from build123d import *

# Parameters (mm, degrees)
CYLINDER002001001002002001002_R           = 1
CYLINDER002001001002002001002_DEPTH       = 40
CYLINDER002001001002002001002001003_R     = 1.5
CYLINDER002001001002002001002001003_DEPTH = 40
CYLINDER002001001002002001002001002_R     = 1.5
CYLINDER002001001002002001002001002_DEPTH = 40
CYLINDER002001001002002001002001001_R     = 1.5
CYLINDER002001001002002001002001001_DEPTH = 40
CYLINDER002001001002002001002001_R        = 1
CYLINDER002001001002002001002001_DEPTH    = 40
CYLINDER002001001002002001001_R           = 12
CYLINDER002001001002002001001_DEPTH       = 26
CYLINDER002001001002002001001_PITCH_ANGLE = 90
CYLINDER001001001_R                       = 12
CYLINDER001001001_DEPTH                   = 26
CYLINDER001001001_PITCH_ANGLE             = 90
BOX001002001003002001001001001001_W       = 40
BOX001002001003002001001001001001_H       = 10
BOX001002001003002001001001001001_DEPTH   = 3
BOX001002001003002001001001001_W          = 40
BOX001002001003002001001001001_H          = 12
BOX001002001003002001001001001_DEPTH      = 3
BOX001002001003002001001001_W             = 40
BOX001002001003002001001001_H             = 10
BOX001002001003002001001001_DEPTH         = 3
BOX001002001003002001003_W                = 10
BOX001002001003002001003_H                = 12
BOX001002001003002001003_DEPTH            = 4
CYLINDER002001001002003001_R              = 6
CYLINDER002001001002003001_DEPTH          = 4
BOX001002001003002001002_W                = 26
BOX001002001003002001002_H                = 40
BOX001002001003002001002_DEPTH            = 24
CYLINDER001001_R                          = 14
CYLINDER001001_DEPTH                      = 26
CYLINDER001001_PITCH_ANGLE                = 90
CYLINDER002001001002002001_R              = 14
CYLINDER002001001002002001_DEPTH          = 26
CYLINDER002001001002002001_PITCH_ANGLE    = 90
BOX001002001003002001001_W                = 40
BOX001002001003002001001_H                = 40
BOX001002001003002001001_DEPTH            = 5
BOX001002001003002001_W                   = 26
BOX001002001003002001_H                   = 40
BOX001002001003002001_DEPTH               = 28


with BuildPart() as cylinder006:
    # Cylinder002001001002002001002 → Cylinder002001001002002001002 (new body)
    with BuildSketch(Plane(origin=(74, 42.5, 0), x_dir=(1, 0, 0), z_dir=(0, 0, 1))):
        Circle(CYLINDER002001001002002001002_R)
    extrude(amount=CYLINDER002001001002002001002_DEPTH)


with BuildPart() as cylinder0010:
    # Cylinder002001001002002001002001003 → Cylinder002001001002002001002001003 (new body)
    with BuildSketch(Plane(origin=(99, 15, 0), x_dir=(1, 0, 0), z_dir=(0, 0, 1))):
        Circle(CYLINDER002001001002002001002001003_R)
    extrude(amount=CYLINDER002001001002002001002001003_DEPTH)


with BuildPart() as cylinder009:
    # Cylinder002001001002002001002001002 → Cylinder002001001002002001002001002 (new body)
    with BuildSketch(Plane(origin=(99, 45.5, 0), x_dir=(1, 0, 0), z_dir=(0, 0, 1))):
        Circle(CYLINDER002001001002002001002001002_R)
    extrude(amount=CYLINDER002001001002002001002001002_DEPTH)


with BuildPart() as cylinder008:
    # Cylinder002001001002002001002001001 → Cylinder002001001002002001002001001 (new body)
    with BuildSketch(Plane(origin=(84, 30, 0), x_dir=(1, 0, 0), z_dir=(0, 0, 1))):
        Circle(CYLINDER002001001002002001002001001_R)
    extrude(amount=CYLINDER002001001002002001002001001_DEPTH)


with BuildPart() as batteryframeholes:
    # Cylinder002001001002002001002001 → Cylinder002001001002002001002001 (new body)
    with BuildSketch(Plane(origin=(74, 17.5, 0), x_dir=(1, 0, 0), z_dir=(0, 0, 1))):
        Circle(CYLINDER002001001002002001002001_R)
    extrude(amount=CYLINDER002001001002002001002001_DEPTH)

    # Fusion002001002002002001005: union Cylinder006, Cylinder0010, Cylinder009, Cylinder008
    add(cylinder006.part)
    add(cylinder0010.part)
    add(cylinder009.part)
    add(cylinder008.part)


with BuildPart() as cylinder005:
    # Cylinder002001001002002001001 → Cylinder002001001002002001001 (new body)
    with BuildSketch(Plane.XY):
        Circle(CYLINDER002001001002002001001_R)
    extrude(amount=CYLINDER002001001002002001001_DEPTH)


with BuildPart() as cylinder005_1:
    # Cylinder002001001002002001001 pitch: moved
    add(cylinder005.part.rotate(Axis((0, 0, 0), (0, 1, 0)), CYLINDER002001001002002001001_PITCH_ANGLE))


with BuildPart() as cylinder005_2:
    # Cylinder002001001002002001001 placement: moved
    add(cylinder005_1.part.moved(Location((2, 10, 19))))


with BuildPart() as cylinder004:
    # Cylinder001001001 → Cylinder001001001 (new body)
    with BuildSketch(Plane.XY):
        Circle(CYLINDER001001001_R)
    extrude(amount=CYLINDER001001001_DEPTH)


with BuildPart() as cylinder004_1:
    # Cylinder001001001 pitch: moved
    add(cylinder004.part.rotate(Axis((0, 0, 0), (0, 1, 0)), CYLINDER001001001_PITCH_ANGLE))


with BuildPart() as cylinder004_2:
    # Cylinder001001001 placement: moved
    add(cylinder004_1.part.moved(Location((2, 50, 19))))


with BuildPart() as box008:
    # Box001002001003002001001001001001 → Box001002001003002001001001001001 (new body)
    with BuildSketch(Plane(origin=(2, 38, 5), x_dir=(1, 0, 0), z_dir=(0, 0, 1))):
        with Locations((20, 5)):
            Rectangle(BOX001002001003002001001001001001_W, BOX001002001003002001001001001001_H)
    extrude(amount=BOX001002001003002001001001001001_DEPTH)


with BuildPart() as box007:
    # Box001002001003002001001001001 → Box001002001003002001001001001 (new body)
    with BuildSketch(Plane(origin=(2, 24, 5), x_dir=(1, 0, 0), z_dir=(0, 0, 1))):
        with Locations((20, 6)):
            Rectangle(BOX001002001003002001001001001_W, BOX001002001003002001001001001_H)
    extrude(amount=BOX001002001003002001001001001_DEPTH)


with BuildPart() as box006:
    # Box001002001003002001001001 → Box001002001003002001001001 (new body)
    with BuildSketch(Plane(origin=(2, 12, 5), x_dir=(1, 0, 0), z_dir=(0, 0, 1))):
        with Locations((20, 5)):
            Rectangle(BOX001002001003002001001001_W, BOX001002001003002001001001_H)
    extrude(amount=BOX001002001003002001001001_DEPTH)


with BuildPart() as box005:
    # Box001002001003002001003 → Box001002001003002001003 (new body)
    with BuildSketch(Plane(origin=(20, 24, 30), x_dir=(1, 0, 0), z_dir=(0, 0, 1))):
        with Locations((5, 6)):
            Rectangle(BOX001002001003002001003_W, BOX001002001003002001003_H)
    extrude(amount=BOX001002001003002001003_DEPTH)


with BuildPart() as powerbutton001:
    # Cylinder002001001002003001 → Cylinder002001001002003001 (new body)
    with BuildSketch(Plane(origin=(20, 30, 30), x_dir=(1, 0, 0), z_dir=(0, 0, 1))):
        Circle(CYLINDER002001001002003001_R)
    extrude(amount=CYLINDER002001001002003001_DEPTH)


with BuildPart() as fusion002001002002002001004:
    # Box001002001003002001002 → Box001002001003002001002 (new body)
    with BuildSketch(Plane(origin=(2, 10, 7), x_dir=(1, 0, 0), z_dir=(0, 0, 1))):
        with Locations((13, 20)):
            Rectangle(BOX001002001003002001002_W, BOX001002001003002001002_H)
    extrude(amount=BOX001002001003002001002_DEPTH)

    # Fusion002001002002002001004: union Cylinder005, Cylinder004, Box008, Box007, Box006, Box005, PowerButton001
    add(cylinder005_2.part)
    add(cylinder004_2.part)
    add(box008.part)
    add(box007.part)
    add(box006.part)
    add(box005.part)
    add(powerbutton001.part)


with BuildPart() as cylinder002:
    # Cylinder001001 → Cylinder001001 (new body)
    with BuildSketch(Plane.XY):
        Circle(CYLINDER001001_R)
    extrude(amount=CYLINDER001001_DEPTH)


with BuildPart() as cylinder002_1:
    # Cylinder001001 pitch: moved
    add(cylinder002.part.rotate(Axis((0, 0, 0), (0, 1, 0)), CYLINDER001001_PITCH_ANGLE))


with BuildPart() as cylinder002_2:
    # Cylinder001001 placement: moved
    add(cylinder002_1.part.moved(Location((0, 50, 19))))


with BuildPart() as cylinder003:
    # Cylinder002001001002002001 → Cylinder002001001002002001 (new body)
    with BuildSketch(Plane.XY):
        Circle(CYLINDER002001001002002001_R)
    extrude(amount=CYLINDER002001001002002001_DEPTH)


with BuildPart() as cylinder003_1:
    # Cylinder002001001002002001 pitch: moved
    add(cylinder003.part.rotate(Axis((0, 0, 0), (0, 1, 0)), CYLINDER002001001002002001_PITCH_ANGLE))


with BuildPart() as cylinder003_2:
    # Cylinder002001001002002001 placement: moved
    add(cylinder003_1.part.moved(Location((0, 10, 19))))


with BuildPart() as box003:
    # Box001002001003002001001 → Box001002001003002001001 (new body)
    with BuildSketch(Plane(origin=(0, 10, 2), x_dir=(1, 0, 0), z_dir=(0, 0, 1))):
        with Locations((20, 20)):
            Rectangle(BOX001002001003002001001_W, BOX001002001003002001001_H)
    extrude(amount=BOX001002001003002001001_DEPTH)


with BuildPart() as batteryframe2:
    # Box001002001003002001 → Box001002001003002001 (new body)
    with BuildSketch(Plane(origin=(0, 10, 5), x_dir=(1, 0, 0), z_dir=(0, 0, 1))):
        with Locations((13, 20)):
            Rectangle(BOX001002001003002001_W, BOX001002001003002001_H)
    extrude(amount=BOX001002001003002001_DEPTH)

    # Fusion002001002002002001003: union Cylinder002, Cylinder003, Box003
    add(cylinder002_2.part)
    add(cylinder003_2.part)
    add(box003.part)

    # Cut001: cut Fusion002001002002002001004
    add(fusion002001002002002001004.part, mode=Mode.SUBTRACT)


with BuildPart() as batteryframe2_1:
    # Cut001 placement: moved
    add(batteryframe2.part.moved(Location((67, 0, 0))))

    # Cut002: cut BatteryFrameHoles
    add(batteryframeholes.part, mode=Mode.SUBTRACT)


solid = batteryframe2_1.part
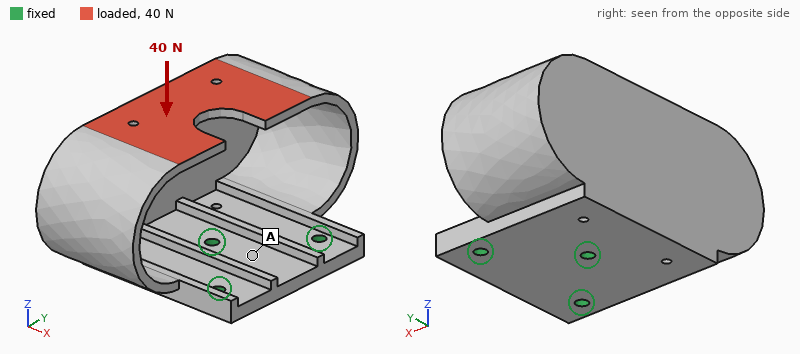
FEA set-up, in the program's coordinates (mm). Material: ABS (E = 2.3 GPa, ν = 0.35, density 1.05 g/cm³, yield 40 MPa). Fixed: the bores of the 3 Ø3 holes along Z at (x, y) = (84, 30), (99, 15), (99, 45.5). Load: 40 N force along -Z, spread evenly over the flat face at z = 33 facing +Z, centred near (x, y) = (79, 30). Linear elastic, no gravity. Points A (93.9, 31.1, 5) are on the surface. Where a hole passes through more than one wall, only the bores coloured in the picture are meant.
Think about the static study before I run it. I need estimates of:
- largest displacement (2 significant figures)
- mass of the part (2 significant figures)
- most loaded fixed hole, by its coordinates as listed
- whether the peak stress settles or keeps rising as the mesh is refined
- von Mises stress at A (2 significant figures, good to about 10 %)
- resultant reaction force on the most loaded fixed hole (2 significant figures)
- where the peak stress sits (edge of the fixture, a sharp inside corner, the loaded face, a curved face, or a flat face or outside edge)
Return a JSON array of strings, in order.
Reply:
["0.98 mm", "15 g", "(84, 30)", "keeps rising", "0.85 MPa", "32 N", "edge of the fixture"]
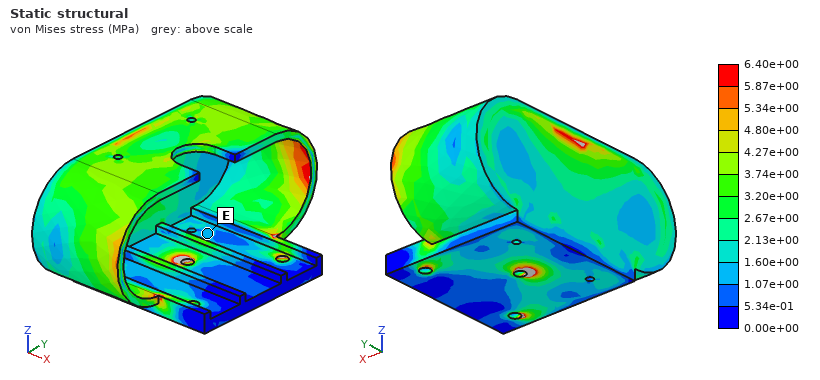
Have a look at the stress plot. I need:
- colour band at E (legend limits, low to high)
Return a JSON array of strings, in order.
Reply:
["1.07e+00 to 1.60e+00 MPa"]
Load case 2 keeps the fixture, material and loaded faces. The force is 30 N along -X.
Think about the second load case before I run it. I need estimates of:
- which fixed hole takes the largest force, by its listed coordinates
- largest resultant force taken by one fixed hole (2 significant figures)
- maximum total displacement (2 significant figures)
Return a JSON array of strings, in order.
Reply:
["(84, 30)", "50 N", "0.96 mm"]
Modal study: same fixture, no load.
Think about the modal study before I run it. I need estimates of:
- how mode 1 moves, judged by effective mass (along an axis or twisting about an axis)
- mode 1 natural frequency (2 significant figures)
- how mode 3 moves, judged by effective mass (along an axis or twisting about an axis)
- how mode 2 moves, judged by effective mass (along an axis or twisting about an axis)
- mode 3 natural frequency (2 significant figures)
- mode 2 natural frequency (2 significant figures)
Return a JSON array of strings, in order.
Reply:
["along Y", "320 Hz", "along Z", "along X", "720 Hz", "470 Hz"]
